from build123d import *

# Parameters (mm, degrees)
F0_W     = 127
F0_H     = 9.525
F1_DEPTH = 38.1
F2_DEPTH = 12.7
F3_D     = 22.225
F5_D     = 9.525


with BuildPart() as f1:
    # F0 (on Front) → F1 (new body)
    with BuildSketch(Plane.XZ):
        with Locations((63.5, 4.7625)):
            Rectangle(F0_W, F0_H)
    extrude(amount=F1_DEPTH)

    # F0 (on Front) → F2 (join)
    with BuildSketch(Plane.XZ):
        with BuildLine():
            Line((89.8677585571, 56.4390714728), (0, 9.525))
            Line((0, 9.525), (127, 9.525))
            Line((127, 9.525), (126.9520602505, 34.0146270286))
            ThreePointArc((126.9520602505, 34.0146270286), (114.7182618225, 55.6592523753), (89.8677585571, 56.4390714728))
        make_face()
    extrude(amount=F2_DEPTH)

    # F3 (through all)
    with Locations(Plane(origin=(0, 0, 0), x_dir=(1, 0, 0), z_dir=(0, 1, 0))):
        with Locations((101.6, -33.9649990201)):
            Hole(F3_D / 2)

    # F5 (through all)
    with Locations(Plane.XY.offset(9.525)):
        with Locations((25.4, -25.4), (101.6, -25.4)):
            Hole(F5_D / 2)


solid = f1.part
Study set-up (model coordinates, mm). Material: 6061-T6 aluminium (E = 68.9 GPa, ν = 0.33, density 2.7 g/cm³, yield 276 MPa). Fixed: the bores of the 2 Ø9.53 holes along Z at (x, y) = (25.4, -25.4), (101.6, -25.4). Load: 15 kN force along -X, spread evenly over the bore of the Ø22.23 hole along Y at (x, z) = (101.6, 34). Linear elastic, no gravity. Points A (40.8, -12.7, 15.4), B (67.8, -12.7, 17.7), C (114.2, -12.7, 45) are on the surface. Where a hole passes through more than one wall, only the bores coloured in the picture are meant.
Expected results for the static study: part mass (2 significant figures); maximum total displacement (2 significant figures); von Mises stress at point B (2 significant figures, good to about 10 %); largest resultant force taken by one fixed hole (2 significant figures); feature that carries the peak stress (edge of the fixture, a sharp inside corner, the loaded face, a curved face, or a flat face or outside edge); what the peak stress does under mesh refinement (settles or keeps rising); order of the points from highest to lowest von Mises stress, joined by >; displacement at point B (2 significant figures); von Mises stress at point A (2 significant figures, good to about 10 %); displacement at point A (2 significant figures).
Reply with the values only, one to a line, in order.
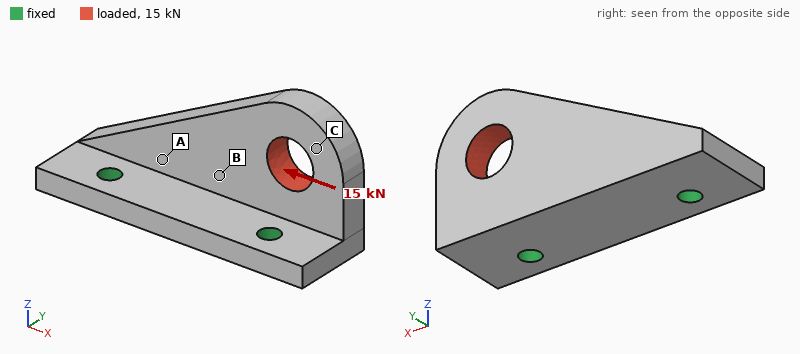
240 g
0.15 mm
37 MPa
9.8 kN
edge of the fixture
keeps rising
A > B > C
0.033 mm
61 MPa
0.036 mm
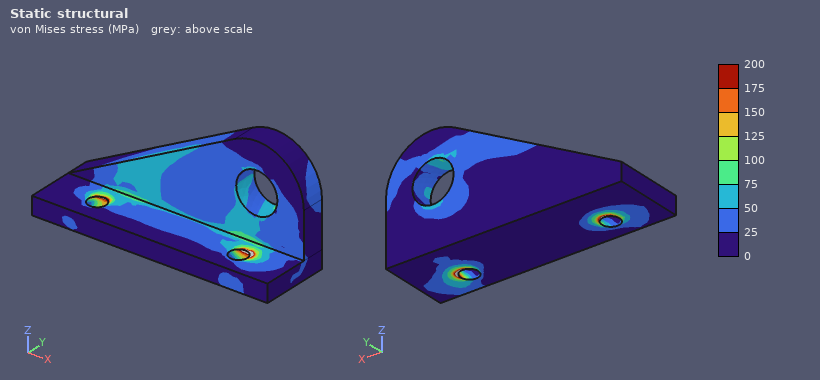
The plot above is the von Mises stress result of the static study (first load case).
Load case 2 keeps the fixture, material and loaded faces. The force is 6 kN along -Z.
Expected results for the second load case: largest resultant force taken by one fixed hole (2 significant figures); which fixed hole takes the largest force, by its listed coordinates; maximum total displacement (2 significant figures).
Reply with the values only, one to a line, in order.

5.8 kN
(101.6, -25.4)
0.19 mm
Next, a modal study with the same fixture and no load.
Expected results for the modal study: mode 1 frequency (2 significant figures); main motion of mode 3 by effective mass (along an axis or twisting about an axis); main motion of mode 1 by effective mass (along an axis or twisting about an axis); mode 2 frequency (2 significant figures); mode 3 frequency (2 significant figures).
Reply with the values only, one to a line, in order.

2300 Hz
along Z
along Y
5200 Hz
6600 Hz
